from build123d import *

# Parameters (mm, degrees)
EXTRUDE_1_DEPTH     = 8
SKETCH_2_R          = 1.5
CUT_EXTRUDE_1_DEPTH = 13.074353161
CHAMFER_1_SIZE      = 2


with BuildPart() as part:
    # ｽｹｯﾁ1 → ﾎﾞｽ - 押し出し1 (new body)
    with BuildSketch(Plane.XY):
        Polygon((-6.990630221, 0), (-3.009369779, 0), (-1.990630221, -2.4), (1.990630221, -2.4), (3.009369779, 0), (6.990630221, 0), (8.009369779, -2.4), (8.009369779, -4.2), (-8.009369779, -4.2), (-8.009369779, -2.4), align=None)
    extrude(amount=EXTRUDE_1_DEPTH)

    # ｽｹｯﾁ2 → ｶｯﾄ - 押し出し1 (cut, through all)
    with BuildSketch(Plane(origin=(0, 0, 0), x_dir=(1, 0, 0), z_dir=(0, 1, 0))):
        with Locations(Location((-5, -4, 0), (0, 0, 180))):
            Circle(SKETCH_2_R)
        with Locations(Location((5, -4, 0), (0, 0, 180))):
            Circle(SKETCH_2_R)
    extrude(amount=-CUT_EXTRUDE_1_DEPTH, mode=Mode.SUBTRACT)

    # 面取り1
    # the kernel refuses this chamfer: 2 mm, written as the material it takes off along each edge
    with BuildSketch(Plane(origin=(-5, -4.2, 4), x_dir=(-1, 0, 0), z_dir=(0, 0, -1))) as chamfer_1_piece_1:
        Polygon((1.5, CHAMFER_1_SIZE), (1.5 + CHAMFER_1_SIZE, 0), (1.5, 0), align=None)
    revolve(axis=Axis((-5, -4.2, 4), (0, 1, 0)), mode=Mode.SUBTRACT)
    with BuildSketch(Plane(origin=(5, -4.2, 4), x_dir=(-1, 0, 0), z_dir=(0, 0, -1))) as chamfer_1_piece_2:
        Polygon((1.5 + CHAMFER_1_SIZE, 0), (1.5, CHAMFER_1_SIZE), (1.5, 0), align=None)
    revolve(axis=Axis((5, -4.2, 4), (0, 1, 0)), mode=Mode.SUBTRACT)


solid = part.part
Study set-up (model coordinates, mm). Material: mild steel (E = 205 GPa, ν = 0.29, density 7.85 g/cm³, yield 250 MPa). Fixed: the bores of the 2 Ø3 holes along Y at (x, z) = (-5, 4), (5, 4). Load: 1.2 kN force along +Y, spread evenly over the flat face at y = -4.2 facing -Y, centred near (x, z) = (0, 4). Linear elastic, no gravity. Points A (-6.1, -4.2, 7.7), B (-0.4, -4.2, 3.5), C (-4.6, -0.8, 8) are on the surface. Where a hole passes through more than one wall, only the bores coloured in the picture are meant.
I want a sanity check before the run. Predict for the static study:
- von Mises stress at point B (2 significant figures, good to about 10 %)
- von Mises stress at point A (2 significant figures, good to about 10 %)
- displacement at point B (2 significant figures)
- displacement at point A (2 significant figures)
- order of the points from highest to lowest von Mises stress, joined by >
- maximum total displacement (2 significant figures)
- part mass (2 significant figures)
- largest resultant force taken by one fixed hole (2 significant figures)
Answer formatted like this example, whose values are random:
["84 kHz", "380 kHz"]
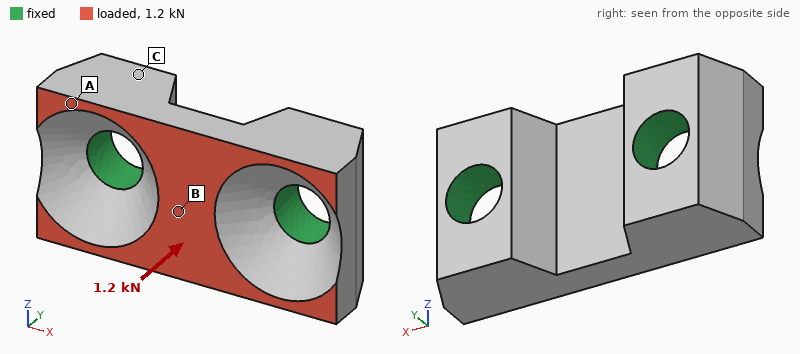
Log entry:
["81 MPa", "33 MPa", "1.9 µm", "1.4 µm", "B > A > C", "3.1 µm", "2.4 g", "660 N"]
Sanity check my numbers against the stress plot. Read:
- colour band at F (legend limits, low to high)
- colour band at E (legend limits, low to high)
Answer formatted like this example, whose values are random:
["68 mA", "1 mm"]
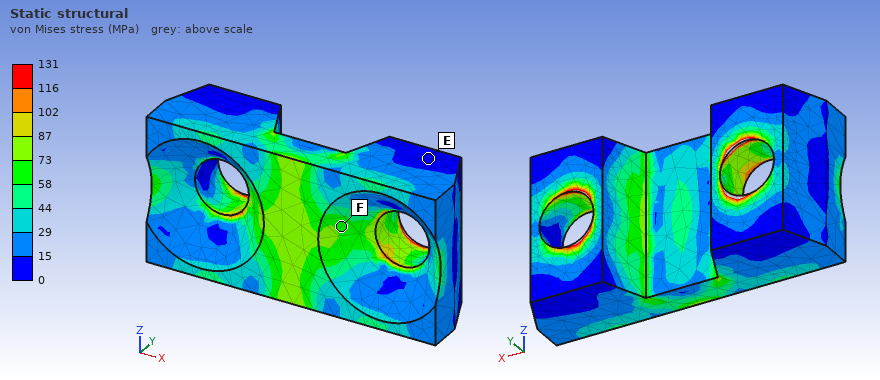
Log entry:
["58 to 73 MPa", "0 to 15 MPa"]
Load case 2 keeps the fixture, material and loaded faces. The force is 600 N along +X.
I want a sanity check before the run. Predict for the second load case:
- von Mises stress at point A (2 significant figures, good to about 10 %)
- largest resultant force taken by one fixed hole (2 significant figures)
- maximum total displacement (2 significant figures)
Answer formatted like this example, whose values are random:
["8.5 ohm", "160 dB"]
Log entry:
["26 MPa", "330 N", "1.3 µm"]
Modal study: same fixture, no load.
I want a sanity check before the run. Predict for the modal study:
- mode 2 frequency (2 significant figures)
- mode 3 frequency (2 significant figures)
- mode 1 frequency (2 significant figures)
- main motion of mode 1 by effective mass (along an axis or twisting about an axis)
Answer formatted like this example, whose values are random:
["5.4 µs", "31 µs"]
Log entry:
["110 kHz", "120 kHz", "85 kHz", "along Z"]
